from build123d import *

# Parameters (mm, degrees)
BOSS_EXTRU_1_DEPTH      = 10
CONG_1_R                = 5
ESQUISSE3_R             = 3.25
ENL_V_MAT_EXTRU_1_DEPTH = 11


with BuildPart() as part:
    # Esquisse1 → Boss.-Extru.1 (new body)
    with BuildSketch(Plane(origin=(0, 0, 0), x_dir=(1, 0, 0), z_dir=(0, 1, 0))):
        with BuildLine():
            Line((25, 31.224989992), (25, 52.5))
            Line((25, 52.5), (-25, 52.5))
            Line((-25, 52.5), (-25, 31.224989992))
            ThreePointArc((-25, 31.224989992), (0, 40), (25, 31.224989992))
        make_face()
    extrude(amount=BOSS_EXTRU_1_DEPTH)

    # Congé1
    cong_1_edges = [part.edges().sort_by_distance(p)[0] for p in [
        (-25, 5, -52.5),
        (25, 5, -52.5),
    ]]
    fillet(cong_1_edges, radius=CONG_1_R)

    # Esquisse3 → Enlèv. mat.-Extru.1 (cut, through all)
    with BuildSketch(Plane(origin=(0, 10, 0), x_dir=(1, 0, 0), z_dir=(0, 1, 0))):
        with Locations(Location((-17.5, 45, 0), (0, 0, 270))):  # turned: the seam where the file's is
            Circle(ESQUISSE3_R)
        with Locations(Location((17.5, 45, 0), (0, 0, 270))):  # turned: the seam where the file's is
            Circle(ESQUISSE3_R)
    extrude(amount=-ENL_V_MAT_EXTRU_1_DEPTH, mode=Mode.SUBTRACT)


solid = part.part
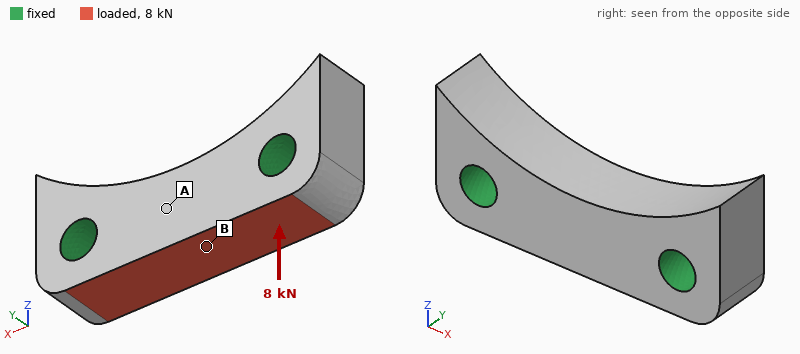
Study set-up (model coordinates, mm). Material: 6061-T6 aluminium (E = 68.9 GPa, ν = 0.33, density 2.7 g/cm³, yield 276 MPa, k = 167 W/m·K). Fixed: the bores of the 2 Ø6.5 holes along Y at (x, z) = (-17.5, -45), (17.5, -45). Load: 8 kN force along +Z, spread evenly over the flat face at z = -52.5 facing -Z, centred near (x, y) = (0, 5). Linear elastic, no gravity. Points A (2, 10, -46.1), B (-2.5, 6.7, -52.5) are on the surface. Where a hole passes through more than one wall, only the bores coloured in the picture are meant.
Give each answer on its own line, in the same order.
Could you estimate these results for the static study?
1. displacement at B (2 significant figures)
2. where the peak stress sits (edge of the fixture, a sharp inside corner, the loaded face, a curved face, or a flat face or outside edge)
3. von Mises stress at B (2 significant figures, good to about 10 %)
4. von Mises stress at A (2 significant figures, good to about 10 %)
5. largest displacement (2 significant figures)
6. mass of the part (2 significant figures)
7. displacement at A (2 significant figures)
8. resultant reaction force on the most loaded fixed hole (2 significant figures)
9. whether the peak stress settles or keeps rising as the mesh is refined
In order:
14 µm
edge of the fixture
41 MPa
13 MPa
15 µm
19 g
14 µm
4.1 kN
keeps rising
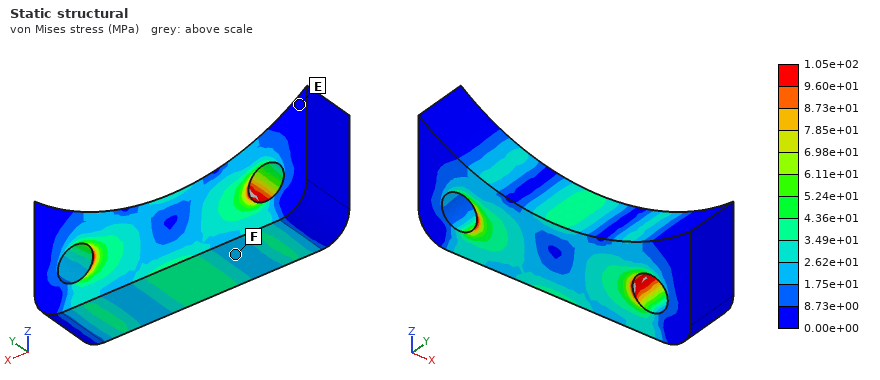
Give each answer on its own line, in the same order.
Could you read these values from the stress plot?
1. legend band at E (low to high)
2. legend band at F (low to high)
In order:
0.00e+00 to 8.73e+00 MPa
1.75e+01 to 2.62e+01 MPa
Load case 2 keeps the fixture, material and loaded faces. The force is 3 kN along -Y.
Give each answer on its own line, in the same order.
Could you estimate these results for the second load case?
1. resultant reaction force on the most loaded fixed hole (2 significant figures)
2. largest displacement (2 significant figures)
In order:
1.5 kN
15 µm
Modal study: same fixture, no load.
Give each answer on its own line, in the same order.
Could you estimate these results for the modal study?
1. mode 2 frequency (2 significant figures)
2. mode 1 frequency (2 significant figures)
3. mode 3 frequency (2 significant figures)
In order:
35 kHz
35 kHz
48 kHz
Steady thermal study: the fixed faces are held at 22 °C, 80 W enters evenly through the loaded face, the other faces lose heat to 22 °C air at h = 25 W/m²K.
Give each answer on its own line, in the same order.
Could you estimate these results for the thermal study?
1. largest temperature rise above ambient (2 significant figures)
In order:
17 K
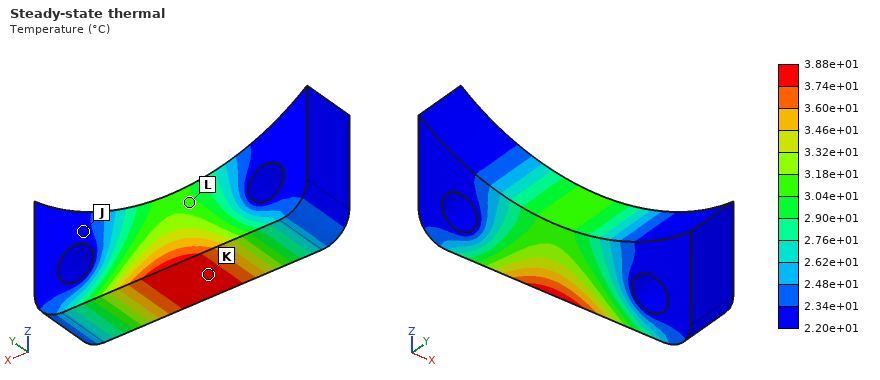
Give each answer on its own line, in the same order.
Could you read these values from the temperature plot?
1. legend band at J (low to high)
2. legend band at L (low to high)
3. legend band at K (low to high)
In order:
2.20e+01 to 2.34e+01 °C
3.04e+01 to 3.18e+01 °C
3.74e+01 to 3.88e+01 °C
